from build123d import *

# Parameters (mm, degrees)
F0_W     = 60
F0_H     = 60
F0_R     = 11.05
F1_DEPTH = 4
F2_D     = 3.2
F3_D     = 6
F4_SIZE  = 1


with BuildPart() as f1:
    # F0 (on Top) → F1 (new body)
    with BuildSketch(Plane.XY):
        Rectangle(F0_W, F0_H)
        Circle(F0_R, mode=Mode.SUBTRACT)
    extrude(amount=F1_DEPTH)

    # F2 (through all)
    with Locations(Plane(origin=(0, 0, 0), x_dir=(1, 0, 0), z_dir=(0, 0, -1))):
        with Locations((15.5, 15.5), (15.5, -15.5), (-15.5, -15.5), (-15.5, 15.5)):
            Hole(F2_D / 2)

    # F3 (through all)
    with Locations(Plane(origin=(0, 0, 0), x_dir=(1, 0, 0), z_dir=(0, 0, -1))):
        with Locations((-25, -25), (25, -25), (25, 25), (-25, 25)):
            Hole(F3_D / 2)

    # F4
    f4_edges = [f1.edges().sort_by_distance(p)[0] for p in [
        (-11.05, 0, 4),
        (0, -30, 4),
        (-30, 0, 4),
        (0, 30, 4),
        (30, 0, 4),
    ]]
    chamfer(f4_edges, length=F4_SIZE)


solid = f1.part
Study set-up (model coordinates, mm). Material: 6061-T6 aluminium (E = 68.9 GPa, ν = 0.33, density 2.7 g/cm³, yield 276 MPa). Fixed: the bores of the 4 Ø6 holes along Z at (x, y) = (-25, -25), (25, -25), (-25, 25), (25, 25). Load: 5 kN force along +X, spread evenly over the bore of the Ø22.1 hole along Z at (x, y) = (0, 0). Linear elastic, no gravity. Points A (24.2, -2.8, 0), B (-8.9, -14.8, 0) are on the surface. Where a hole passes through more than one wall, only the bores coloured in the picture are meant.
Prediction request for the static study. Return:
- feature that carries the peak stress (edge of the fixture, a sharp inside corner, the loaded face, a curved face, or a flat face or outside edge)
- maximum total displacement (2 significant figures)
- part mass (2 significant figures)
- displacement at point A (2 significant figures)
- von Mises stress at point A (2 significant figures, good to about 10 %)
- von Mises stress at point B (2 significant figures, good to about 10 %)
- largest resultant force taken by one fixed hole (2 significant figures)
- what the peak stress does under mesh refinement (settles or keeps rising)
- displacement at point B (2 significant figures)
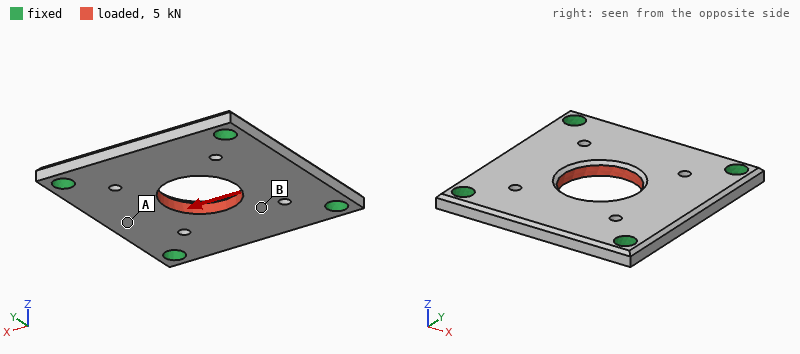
edge of the fixture
13 µm
33 g
11 µm
6.5 MPa
23 MPa
1.4 kN
keeps rising
7.0 µm
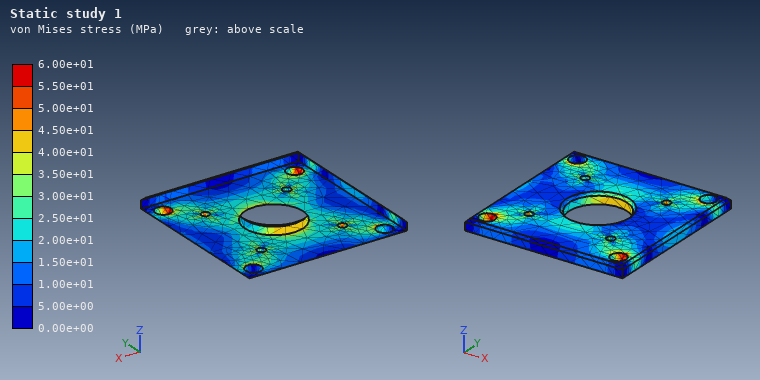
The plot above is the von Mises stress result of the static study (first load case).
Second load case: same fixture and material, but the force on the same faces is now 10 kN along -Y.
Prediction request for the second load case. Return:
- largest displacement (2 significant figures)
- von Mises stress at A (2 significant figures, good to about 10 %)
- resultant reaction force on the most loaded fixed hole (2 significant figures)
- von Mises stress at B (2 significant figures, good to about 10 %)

27 µm
21 MPa
2.8 kN
52 MPa
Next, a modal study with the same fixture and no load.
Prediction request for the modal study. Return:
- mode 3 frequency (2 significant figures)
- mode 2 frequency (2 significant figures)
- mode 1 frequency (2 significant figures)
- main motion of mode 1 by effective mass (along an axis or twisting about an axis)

9600 Hz
9600 Hz
6600 Hz
along Z
